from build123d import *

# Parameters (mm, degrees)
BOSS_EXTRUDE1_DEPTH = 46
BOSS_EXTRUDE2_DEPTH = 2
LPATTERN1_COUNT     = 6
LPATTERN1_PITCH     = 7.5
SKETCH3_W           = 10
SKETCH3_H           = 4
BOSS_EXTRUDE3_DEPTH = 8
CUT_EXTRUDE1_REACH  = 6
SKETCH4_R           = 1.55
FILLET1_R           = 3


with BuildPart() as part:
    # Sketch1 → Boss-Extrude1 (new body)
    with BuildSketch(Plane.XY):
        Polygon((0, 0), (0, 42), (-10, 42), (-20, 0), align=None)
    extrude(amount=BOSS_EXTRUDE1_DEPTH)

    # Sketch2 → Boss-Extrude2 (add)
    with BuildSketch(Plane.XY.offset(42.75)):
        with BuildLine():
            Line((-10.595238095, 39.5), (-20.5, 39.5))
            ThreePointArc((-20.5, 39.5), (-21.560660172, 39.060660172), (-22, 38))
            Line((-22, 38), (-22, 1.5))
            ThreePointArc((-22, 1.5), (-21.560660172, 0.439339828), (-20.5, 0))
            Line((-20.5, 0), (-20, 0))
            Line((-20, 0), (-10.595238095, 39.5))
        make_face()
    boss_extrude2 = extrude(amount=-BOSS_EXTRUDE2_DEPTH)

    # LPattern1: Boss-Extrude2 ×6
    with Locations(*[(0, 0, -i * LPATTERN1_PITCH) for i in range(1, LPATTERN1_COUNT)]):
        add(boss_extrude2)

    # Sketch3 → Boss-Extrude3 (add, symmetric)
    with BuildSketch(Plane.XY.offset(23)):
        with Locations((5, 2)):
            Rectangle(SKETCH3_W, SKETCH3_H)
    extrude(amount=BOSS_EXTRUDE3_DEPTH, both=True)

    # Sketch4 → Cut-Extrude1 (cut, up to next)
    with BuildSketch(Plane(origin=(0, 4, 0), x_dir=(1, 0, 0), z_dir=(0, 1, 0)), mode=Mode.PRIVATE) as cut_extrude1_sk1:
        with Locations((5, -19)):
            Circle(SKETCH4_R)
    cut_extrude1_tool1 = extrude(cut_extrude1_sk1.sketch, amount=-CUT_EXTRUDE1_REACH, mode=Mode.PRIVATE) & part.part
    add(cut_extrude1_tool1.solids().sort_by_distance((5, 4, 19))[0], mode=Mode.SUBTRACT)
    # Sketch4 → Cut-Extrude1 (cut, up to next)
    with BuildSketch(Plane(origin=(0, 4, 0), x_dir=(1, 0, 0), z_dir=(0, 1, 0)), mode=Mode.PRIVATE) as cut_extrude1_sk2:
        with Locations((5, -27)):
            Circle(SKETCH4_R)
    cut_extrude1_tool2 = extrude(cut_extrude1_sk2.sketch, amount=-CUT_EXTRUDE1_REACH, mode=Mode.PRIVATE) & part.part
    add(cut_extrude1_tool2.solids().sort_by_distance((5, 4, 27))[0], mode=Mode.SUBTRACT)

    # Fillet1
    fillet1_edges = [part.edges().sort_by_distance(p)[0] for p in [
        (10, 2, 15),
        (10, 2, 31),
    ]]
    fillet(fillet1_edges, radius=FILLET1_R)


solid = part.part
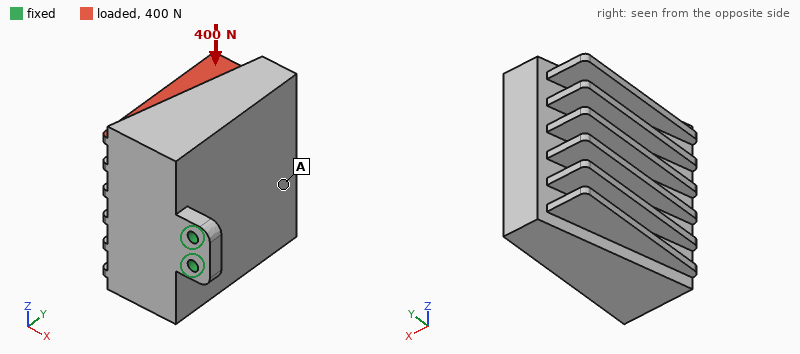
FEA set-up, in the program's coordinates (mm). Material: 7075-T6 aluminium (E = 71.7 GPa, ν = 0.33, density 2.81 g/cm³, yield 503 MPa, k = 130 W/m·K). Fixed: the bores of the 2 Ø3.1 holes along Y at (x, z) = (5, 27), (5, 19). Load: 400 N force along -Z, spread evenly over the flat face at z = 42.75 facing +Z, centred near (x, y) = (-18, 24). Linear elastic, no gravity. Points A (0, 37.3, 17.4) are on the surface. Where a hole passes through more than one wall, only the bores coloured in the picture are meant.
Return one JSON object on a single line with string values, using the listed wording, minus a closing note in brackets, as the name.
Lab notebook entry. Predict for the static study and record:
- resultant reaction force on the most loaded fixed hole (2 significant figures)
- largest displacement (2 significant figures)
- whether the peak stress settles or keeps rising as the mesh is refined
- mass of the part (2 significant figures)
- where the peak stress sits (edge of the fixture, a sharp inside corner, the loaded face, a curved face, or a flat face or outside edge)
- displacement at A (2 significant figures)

{"resultant reaction force on the most loaded fixed hole": "1.2 kN", "largest displacement": "0.15 mm", "whether the peak stress settles or keeps rising as the mesh is refined": "keeps rising", "mass of the part": "92 g", "where the peak stress sits": "edge of the fixture", "displacement at A": "0.086 mm"}
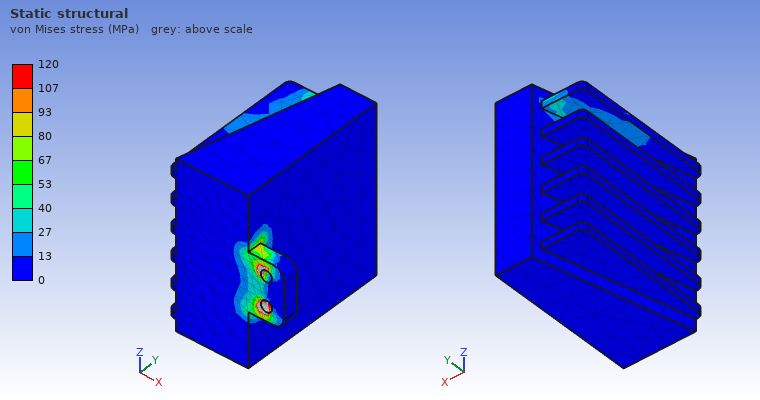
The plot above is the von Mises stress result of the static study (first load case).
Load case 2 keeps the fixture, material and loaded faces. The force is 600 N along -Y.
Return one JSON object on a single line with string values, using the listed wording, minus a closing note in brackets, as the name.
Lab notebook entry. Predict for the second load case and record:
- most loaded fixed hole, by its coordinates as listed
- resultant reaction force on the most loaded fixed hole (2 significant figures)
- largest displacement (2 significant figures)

{"most loaded fixed hole, by its coordinates as listed": "(5, 27)", "resultant reaction force on the most loaded fixed hole": "1.3 kN", "largest displacement": "0.56 mm"}
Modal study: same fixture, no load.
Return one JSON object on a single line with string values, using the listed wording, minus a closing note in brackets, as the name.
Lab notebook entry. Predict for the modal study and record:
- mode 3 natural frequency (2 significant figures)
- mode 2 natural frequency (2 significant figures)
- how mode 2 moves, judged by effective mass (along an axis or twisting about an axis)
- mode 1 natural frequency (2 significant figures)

{"mode 3 natural frequency": "3100 Hz", "mode 2 natural frequency": "1300 Hz", "how mode 2 moves, judged by effective mass": "along Z", "mode 1 natural frequency": "710 Hz"}
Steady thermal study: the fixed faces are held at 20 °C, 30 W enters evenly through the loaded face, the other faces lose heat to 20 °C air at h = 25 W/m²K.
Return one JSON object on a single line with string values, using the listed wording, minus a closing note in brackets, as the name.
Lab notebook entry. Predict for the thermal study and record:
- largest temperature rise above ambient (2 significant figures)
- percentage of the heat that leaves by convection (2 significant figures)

{"largest temperature rise above ambient": "56 K", "percentage of the heat that leaves by convection": "20 %"}
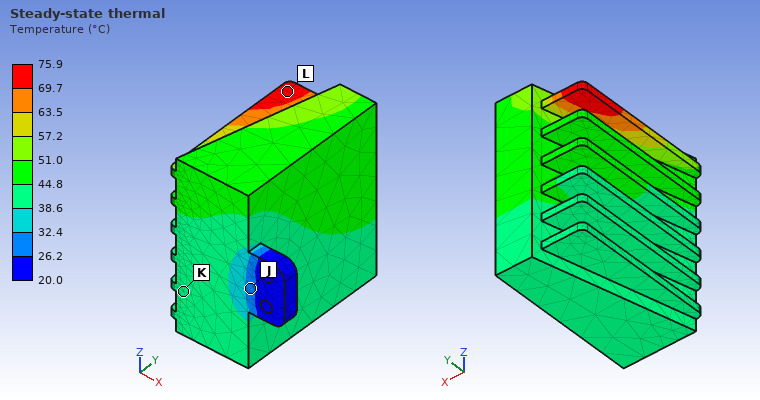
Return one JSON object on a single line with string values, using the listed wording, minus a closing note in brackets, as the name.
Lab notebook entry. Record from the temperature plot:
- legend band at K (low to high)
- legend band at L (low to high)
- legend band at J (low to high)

{"legend band at K": "38.6 to 44.8 °C", "legend band at L": "69.7 to 75.9 °C", "legend band at J": "26.2 to 32.4 °C"}
